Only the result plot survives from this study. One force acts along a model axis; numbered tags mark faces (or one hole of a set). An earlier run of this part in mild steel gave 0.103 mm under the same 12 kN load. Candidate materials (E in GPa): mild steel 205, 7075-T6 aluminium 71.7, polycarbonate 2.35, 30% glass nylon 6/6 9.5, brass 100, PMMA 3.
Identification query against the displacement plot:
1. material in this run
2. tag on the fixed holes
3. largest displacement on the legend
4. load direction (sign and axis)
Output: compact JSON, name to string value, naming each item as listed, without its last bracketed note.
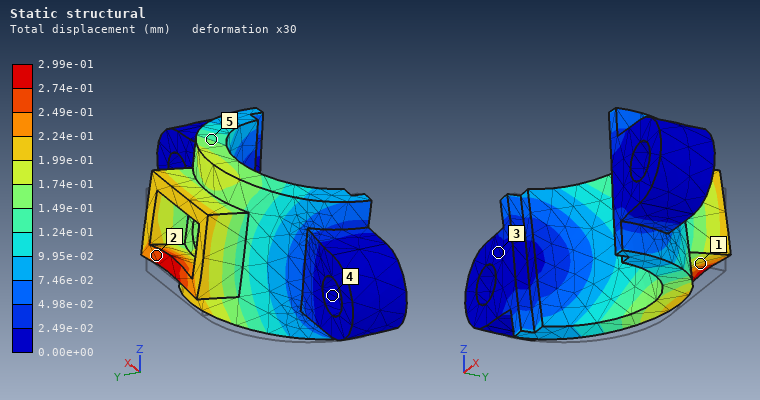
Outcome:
{"material in this run": "7075-T6 aluminium", "tag on the fixed holes": "4", "largest displacement on the legend": "2.99e-01 mm", "load direction": "+Z"}
